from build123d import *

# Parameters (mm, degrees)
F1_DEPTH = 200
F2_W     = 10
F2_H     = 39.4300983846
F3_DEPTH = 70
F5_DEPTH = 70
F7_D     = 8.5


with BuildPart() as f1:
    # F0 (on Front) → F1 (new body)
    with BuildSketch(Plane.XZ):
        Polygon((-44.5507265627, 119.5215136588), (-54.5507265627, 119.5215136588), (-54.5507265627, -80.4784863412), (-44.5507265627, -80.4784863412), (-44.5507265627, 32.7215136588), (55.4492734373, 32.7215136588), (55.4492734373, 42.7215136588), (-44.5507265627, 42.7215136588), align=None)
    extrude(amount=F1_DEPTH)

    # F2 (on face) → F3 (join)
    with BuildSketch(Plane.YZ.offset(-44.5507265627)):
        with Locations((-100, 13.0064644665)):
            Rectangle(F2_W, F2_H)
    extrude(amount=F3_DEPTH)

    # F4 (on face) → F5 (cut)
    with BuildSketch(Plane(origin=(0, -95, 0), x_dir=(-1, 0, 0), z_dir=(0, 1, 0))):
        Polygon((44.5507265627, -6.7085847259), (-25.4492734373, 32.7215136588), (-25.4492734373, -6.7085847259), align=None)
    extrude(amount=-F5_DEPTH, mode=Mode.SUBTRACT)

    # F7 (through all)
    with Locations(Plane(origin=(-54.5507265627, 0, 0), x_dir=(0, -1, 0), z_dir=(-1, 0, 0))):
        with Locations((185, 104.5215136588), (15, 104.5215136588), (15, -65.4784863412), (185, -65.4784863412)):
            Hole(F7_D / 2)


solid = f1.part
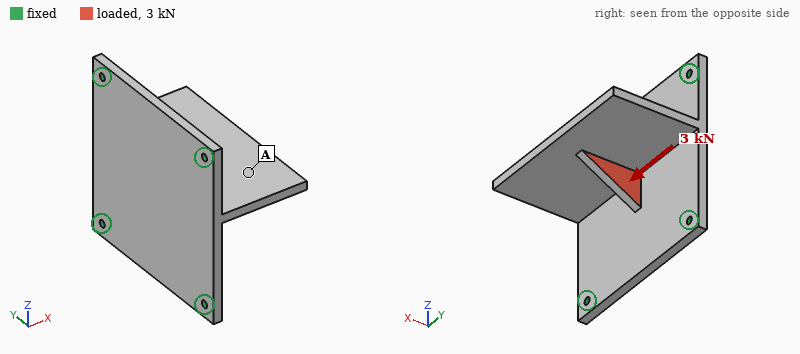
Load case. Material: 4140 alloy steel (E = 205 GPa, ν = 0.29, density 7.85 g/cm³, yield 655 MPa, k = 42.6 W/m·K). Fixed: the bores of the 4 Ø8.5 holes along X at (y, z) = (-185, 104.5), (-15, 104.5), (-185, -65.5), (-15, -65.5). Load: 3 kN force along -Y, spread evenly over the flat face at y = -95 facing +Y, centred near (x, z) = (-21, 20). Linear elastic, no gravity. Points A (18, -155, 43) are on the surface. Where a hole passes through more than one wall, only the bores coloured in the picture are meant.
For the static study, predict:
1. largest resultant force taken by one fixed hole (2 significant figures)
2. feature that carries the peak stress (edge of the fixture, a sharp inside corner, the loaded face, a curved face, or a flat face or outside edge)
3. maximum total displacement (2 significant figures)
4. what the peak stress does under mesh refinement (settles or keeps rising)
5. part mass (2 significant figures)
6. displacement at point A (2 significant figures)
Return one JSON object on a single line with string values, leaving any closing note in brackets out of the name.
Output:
{"largest resultant force taken by one fixed hole": "990 N", "feature that carries the peak stress": "edge of the fixture", "maximum total displacement": "19 µm", "what the peak stress does under mesh refinement": "keeps rising", "part mass": "4.8 kg", "displacement at point A": "12 µm"}
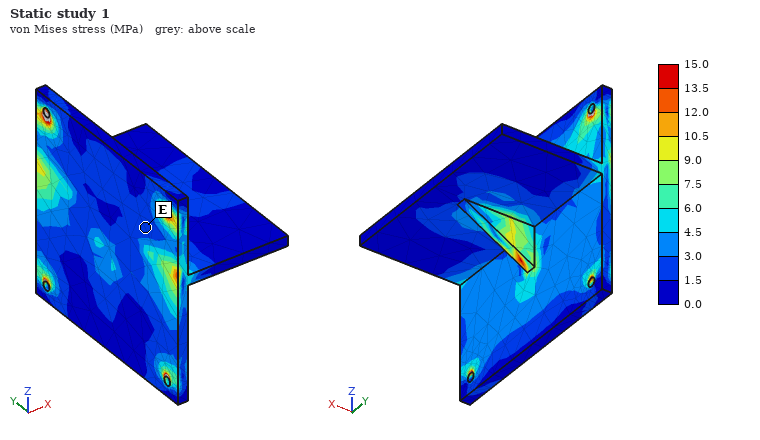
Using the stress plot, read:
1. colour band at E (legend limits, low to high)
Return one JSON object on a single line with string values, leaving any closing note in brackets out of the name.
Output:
{"colour band at E": "1.5 to 3.0 MPa"}
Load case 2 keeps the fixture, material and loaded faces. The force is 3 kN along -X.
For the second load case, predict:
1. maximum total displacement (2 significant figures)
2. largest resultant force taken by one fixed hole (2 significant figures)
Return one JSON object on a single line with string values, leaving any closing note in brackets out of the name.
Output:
{"maximum total displacement": "41 µm", "largest resultant force taken by one fixed hole": "850 N"}
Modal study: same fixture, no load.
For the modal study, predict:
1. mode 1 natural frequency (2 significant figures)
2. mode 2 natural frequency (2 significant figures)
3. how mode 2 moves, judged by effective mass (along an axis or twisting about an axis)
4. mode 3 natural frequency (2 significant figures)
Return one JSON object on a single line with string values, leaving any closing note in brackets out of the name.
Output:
{"mode 1 natural frequency": "820 Hz", "mode 2 natural frequency": "950 Hz", "how mode 2 moves, judged by effective mass": "along X", "mode 3 natural frequency": "1000 Hz"}
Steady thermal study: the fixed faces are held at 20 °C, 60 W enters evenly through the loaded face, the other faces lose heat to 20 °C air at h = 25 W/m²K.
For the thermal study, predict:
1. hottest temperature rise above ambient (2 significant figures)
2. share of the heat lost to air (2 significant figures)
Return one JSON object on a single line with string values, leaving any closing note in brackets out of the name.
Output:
{"hottest temperature rise above ambient": "56 K", "share of the heat lost to air": "70 %"}
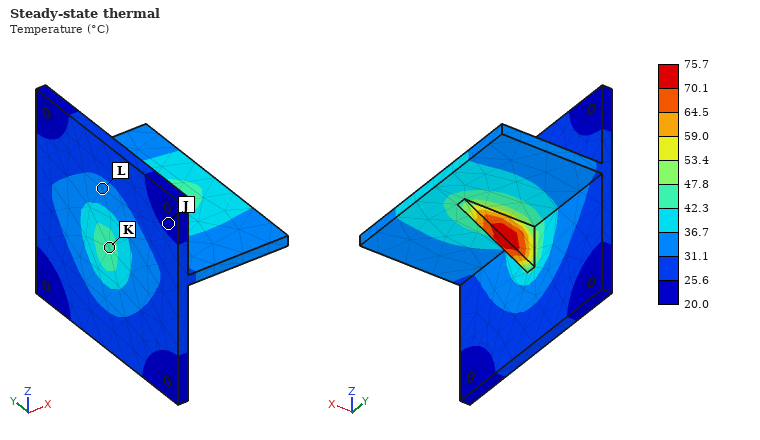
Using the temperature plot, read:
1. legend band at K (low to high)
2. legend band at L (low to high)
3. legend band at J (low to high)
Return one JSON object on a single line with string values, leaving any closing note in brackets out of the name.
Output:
{"legend band at K": "42.3 to 47.8 °C", "legend band at L": "31.1 to 36.7 °C", "legend band at J": "20.0 to 25.6 °C"}
